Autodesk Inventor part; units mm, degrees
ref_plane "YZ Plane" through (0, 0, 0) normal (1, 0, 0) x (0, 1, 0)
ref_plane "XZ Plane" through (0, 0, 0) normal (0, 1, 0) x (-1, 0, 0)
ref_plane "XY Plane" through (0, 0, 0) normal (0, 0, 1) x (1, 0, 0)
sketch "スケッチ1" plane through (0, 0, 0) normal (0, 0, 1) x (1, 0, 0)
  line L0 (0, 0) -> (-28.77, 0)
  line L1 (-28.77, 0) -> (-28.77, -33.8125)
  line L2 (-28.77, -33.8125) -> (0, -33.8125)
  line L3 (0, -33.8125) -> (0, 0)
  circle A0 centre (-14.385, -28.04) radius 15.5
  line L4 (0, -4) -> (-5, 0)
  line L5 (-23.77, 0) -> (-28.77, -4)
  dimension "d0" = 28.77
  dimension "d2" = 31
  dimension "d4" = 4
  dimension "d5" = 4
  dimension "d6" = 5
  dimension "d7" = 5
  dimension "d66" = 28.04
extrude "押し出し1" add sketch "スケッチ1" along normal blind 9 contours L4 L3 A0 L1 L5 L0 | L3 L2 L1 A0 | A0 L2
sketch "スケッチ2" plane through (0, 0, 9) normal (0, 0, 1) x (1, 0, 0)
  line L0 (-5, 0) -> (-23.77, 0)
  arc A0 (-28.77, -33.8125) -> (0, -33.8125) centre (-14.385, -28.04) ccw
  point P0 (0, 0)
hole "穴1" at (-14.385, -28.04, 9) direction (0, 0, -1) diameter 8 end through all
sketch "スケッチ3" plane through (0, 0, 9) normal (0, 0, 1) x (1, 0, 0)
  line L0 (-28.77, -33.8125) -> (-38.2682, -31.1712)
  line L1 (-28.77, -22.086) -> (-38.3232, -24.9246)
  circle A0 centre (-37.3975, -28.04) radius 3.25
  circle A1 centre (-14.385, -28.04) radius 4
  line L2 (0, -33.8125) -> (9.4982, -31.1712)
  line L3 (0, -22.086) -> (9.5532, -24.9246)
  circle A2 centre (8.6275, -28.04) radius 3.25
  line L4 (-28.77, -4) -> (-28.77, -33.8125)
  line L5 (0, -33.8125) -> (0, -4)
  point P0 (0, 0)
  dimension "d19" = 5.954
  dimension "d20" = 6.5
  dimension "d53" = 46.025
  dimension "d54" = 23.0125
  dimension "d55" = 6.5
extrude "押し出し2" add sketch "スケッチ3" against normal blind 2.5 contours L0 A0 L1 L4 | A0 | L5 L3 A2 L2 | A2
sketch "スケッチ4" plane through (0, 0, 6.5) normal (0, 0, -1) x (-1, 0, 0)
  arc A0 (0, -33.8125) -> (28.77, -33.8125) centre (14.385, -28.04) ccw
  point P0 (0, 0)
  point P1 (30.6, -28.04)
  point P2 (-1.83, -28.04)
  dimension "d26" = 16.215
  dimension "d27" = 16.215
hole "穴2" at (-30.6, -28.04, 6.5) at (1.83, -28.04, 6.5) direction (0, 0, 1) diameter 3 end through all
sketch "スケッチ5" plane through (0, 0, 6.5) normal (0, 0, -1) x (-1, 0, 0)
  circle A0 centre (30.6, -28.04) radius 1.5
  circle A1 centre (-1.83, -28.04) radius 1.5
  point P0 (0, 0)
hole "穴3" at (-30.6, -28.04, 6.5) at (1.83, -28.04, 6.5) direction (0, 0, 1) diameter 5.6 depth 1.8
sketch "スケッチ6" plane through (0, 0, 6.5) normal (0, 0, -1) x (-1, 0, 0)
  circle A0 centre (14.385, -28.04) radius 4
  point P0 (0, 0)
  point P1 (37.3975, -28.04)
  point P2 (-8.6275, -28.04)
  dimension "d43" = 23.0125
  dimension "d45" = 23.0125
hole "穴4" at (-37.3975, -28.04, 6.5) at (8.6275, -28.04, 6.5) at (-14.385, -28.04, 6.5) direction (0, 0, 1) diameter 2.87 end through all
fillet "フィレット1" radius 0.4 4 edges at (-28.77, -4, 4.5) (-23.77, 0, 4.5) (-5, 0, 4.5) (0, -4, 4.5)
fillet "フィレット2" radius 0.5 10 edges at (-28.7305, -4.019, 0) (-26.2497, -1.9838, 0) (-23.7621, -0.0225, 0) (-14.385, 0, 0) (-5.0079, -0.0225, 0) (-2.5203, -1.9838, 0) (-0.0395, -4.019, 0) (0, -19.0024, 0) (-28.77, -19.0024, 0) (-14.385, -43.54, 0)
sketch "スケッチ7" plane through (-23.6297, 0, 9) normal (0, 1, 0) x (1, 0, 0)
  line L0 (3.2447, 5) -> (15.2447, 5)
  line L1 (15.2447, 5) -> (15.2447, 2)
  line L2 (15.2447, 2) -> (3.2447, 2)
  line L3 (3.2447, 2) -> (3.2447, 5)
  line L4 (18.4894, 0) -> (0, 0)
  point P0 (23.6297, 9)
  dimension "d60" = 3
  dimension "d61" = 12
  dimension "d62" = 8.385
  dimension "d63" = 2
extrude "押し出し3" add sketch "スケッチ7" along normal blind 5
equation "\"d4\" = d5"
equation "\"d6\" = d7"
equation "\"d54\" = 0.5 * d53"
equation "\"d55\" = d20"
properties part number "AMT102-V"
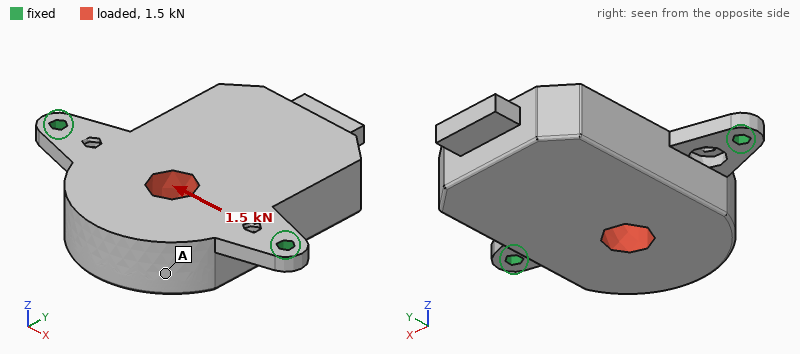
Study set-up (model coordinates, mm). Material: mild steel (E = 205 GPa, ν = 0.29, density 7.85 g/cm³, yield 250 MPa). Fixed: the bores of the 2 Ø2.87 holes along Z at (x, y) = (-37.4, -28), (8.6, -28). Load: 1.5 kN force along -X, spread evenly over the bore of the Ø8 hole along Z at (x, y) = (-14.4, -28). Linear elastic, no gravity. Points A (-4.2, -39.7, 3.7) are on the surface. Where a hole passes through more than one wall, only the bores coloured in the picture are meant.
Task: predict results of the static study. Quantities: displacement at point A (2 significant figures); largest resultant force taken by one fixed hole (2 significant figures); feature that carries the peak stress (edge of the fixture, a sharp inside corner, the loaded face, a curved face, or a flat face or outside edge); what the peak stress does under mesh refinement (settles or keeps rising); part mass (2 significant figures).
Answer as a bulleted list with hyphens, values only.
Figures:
- 5.0 µm
- 760 N
- edge of the fixture
- keeps rising
- 82 g
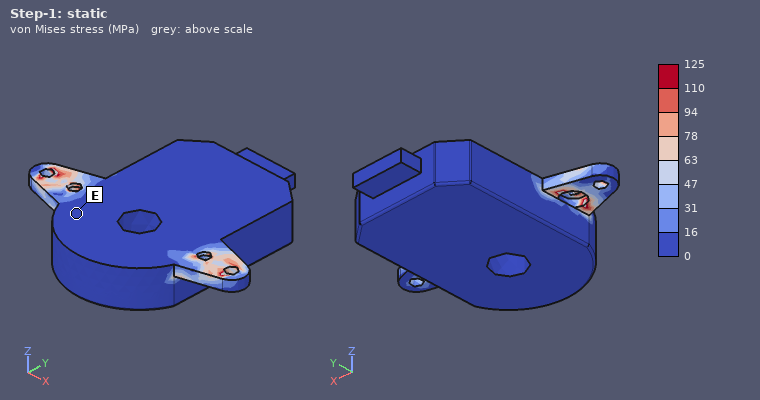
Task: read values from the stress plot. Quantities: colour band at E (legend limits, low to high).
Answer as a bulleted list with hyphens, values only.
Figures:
- 0 to 16 MPa
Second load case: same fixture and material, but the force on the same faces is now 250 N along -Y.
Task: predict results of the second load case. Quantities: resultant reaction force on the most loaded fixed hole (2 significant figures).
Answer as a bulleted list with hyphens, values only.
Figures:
- 130 N
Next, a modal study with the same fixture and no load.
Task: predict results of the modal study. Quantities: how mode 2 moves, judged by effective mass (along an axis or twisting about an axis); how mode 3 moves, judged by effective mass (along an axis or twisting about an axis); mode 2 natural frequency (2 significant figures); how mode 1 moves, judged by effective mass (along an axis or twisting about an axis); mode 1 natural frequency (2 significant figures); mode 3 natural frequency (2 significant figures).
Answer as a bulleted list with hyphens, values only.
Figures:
- along Z
- along X
- 4300 Hz
- along Z
- 1000 Hz
- 7000 Hz
